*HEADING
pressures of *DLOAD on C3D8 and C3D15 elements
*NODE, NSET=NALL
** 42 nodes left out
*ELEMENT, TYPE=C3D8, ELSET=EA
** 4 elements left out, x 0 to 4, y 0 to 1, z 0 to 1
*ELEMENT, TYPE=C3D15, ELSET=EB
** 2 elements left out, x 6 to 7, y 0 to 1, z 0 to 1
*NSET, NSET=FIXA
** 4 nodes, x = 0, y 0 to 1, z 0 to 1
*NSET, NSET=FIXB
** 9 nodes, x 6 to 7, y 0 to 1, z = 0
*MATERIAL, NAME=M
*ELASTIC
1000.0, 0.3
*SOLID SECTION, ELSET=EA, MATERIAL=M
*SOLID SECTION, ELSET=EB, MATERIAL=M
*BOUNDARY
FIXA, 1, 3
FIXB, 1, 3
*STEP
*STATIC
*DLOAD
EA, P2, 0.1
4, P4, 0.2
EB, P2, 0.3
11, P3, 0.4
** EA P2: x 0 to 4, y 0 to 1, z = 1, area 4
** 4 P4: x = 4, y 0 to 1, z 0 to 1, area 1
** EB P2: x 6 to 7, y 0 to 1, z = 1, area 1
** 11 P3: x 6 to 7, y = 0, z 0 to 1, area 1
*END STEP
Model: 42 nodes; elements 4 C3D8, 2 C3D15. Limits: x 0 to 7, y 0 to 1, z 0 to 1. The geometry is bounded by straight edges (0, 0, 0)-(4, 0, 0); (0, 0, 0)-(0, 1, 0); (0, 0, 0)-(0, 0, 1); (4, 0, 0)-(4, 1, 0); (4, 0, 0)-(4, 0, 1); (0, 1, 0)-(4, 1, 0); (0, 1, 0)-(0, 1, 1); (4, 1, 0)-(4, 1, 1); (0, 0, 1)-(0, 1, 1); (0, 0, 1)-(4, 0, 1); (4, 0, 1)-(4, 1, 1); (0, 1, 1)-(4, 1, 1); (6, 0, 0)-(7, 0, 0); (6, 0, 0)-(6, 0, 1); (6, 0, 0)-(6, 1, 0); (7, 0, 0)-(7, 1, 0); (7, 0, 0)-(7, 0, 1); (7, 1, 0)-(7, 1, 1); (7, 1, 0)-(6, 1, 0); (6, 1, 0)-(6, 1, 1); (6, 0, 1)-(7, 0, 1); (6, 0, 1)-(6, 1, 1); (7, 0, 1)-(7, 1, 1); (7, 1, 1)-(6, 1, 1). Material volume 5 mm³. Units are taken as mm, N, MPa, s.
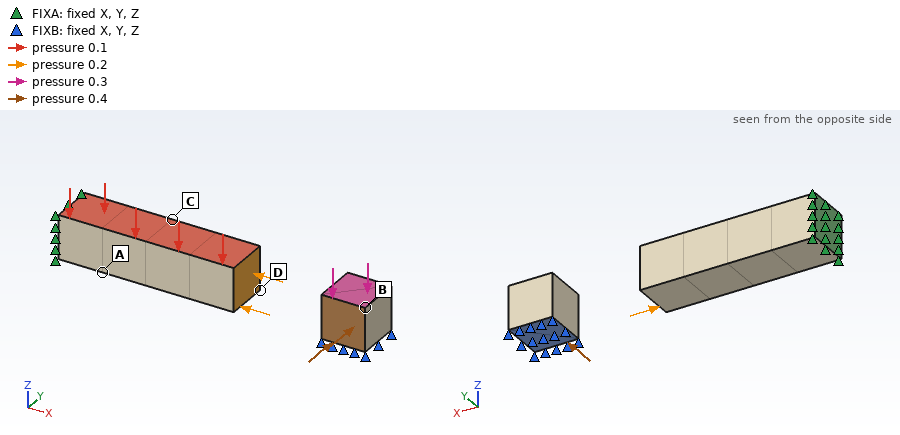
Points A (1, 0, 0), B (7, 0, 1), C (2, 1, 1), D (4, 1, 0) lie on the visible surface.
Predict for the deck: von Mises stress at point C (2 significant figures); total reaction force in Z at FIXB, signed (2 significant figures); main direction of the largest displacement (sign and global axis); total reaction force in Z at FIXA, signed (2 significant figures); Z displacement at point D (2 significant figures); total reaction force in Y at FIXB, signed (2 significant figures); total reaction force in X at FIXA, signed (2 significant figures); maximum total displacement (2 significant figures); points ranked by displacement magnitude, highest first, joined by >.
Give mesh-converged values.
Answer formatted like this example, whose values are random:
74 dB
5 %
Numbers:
1.0 MPa
0.30 N
-Z
0.40 N
-0.040 mm
-0.40 N
0.20 N
0.040 mm
D > C > A > B
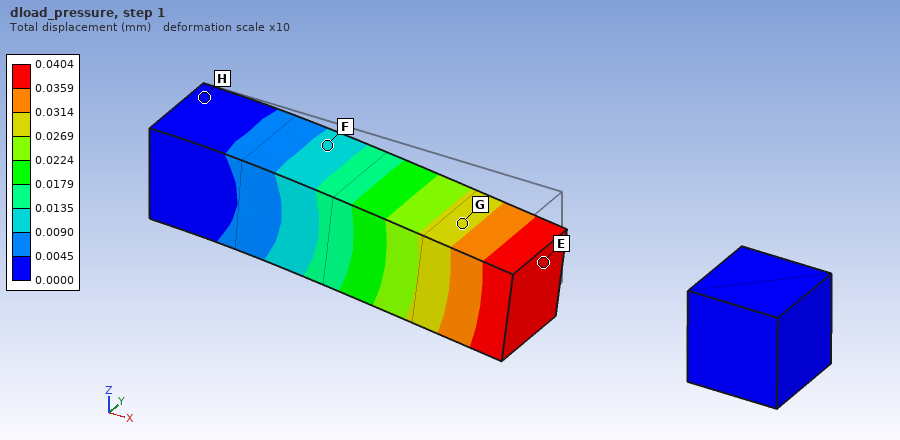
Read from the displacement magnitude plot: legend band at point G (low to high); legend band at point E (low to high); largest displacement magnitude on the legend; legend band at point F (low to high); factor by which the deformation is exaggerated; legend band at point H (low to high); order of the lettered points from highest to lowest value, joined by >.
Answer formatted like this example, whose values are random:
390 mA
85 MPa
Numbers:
0.0269 to 0.0314 mm
0.0359 to 0.0404 mm
0.0404 mm
0.0090 to 0.0135 mm
10
0.0000 to 0.0045 mm
E > G > F > H
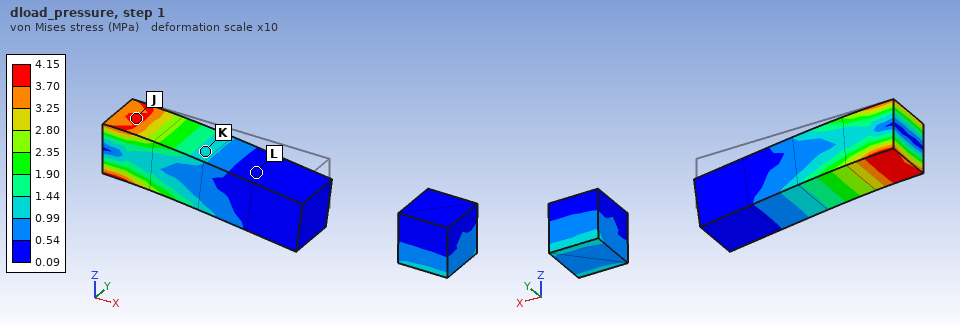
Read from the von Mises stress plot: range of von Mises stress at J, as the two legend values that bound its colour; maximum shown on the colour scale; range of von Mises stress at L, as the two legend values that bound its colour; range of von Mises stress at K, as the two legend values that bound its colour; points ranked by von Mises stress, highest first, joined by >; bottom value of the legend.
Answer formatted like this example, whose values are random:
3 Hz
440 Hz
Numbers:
3.70 to 4.15 MPa
4.15 MPa
0.09 to 0.54 MPa
0.99 to 1.44 MPa
J > K > L
0.09 MPa
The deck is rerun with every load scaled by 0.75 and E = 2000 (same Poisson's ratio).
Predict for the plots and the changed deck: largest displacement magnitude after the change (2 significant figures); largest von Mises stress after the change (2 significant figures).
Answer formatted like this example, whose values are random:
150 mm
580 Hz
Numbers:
0.015 mm
3.1 MPa
